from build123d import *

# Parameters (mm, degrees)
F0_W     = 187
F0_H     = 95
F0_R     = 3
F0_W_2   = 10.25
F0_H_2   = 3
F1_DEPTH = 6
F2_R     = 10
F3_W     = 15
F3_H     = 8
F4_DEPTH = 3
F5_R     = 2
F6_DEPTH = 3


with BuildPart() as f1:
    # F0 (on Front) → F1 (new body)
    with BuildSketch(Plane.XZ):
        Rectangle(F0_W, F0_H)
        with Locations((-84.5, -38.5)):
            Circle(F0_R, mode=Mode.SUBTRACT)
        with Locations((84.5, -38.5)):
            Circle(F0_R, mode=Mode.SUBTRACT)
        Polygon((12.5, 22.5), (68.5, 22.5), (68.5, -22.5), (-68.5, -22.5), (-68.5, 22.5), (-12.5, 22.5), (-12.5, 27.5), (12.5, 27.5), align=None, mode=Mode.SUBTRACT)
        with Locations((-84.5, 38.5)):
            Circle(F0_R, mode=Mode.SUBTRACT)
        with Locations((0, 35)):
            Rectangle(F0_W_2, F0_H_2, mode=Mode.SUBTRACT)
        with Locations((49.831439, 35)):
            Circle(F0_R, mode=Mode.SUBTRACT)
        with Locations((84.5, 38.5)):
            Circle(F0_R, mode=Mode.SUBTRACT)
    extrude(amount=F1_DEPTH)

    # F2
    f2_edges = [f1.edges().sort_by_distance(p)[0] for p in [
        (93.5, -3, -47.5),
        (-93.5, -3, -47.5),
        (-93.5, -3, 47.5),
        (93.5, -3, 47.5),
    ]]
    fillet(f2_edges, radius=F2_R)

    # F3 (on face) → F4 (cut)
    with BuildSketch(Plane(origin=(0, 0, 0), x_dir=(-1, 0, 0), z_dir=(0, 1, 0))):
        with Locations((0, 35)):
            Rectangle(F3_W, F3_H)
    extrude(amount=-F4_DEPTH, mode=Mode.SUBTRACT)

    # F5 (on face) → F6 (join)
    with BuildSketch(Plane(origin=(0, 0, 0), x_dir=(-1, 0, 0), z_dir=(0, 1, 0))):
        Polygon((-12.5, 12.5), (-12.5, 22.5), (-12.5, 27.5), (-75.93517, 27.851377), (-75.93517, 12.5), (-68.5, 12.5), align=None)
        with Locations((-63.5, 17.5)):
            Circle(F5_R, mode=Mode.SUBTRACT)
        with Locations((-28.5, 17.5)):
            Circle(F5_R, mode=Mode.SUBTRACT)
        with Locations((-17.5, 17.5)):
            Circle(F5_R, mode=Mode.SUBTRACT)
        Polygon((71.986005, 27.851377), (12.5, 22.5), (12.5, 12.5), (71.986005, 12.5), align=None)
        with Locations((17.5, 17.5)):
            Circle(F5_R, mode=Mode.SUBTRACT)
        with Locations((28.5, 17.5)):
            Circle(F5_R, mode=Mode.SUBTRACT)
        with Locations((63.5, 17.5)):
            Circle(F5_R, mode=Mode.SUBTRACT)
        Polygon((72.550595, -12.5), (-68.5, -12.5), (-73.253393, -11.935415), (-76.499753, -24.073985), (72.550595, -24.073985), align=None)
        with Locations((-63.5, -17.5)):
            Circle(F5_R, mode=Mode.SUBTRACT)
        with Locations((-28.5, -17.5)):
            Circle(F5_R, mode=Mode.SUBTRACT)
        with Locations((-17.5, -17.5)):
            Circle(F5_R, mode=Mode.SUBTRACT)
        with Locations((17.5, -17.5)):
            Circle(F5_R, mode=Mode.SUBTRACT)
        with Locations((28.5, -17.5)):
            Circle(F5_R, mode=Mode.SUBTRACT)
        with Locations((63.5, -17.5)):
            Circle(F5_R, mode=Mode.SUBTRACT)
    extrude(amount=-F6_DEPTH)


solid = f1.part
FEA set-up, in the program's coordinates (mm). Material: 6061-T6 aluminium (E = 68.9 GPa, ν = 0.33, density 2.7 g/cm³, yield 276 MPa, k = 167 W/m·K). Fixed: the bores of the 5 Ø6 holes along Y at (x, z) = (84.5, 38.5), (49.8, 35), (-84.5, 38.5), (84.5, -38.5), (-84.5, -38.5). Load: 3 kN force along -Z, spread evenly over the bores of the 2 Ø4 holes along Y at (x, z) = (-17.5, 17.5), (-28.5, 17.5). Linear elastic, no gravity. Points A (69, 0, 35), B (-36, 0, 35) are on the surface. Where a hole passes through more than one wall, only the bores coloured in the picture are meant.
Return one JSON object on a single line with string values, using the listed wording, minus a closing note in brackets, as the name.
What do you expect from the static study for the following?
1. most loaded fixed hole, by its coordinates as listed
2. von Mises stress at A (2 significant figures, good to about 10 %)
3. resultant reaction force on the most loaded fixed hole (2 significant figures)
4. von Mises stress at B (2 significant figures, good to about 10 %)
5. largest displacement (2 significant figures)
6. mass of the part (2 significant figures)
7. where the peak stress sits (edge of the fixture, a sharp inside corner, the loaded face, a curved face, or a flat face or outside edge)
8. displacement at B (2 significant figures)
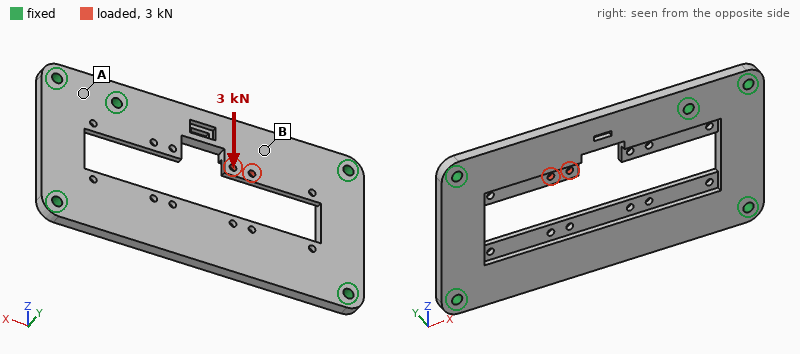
{"most loaded fixed hole, by its coordinates as listed": "(49.8, 35)", "von Mises stress at A": "12 MPa", "resultant reaction force on the most loaded fixed hole": "2.1 kN", "von Mises stress at B": "45 MPa", "largest displacement": "0.19 mm", "mass of the part": "200 g", "where the peak stress sits": "a flat face or outside edge", "displacement at B": "0.092 mm"}
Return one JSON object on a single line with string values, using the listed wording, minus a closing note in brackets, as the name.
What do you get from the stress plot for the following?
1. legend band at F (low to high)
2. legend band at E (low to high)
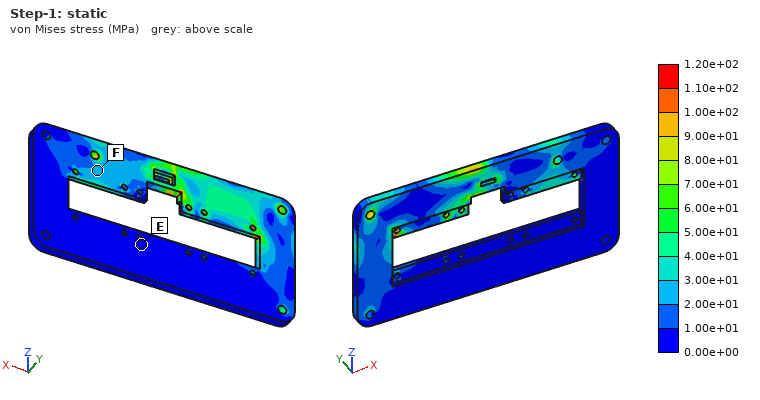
{"legend band at F": "2.00e+01 to 3.00e+01 MPa", "legend band at E": "0.00e+00 to 1.00e+01 MPa"}
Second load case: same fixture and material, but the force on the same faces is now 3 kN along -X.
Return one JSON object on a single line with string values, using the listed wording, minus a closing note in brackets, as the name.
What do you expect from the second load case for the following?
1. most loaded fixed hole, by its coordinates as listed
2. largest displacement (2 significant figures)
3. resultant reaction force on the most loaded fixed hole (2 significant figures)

{"most loaded fixed hole, by its coordinates as listed": "(-84.5, 38.5)", "largest displacement": "64 µm", "resultant reaction force on the most loaded fixed hole": "2.2 kN"}
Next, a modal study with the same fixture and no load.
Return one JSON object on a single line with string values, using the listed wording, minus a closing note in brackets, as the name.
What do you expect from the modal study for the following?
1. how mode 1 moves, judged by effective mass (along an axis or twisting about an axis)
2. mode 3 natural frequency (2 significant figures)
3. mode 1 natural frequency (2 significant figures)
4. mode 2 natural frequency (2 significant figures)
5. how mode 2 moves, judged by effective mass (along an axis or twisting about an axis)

{"how mode 1 moves, judged by effective mass": "along Y", "mode 3 natural frequency": "2900 Hz", "mode 1 natural frequency": "1100 Hz", "mode 2 natural frequency": "1700 Hz", "how mode 2 moves, judged by effective mass": "along Y"}
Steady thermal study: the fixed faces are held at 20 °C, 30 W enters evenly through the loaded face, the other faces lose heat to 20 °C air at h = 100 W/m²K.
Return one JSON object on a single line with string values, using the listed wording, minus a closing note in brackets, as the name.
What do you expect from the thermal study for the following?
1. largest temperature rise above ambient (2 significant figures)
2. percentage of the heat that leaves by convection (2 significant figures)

{"largest temperature rise above ambient": "51 K", "percentage of the heat that leaves by convection": "45 %"}
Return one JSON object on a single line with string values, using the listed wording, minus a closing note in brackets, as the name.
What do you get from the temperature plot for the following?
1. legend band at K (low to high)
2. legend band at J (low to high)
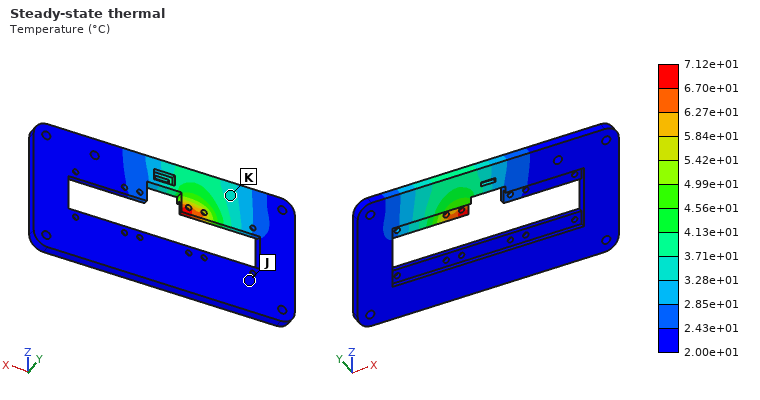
{"legend band at K": "3.28e+01 to 3.71e+01 °C", "legend band at J": "2.00e+01 to 2.43e+01 °C"}
